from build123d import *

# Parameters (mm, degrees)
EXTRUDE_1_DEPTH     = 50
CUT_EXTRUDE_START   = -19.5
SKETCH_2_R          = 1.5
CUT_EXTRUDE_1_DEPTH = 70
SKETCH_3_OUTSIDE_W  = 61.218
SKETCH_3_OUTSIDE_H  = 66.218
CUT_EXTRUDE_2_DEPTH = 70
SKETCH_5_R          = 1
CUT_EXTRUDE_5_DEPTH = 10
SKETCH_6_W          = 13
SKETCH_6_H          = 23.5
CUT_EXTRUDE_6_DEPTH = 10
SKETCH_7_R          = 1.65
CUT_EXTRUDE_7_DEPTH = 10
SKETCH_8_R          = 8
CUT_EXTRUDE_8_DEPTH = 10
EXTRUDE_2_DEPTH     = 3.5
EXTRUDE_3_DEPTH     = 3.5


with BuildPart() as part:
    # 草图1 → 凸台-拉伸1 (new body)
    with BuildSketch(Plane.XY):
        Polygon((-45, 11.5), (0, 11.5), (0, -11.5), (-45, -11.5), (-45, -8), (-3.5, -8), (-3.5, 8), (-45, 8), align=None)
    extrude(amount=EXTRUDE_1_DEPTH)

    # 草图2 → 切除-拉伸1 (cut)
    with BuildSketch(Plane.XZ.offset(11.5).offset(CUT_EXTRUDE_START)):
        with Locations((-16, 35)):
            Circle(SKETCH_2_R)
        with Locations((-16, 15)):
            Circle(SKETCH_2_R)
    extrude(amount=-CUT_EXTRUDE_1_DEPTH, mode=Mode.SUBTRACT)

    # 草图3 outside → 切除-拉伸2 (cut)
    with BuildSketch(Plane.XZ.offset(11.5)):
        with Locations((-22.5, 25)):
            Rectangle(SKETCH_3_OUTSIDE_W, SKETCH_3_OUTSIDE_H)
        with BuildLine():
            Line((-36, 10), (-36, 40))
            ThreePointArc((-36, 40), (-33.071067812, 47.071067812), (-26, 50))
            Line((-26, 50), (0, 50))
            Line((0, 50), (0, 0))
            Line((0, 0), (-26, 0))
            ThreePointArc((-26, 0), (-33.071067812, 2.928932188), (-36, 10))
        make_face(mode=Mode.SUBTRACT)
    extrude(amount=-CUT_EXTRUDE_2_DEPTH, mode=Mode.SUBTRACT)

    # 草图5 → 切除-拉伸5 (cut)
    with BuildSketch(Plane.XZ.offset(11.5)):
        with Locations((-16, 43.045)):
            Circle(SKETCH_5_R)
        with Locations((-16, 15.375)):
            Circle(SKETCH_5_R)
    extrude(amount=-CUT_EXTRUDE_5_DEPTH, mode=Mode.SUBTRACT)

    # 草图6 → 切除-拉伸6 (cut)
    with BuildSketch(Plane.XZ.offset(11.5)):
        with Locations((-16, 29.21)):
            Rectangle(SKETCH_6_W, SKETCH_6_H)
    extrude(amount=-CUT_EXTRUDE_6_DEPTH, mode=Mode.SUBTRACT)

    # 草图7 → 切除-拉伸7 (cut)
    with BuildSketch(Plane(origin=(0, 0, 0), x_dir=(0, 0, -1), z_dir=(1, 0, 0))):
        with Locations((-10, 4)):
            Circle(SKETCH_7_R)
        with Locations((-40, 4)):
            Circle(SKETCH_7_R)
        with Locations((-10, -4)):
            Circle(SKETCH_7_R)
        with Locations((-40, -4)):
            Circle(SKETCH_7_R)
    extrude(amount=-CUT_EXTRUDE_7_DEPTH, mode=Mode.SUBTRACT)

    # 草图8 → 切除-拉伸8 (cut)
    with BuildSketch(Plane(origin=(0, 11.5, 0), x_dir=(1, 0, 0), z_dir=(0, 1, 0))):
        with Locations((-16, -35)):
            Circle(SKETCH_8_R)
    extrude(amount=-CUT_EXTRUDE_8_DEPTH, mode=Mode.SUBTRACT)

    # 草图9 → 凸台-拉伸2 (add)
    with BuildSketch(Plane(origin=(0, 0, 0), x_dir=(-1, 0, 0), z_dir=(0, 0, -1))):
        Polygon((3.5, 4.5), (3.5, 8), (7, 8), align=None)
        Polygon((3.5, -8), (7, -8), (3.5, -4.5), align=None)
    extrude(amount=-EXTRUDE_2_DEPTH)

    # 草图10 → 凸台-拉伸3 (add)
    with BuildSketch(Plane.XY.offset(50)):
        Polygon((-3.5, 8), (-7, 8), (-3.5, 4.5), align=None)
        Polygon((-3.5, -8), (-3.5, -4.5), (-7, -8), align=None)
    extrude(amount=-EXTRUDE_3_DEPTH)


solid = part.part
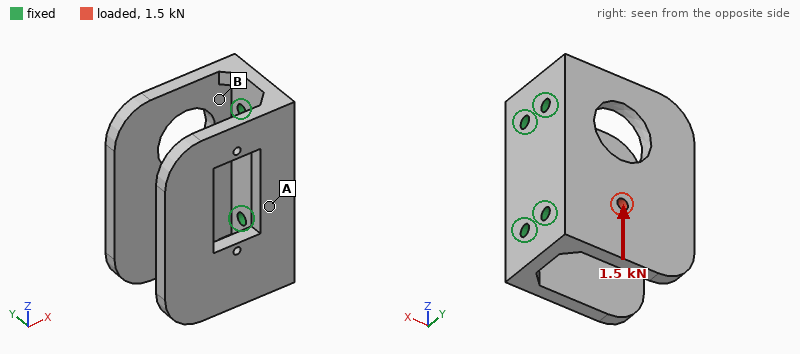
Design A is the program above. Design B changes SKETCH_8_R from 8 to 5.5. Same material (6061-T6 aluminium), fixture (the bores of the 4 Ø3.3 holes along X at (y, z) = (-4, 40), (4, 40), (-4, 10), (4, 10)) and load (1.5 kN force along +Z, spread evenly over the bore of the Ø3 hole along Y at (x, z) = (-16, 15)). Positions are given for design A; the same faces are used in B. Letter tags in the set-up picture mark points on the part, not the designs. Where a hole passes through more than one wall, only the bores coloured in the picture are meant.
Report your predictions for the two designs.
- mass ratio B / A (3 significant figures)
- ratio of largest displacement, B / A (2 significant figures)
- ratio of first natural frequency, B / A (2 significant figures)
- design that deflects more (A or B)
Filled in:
1.03
0.88
1.0
A
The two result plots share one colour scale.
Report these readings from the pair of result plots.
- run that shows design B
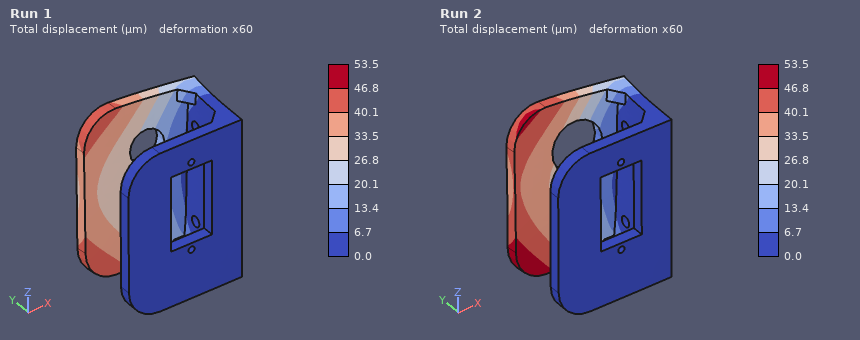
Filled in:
Run 1
